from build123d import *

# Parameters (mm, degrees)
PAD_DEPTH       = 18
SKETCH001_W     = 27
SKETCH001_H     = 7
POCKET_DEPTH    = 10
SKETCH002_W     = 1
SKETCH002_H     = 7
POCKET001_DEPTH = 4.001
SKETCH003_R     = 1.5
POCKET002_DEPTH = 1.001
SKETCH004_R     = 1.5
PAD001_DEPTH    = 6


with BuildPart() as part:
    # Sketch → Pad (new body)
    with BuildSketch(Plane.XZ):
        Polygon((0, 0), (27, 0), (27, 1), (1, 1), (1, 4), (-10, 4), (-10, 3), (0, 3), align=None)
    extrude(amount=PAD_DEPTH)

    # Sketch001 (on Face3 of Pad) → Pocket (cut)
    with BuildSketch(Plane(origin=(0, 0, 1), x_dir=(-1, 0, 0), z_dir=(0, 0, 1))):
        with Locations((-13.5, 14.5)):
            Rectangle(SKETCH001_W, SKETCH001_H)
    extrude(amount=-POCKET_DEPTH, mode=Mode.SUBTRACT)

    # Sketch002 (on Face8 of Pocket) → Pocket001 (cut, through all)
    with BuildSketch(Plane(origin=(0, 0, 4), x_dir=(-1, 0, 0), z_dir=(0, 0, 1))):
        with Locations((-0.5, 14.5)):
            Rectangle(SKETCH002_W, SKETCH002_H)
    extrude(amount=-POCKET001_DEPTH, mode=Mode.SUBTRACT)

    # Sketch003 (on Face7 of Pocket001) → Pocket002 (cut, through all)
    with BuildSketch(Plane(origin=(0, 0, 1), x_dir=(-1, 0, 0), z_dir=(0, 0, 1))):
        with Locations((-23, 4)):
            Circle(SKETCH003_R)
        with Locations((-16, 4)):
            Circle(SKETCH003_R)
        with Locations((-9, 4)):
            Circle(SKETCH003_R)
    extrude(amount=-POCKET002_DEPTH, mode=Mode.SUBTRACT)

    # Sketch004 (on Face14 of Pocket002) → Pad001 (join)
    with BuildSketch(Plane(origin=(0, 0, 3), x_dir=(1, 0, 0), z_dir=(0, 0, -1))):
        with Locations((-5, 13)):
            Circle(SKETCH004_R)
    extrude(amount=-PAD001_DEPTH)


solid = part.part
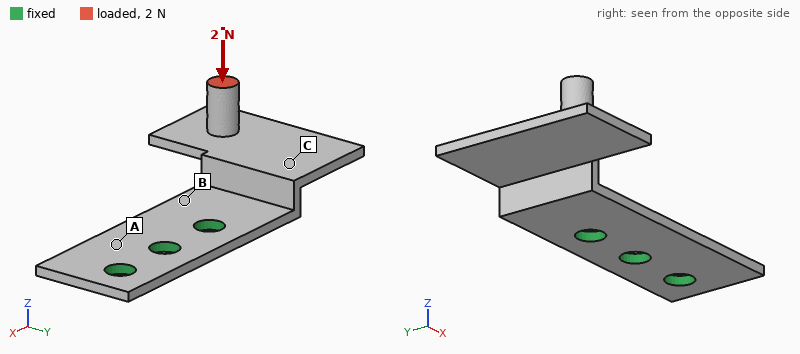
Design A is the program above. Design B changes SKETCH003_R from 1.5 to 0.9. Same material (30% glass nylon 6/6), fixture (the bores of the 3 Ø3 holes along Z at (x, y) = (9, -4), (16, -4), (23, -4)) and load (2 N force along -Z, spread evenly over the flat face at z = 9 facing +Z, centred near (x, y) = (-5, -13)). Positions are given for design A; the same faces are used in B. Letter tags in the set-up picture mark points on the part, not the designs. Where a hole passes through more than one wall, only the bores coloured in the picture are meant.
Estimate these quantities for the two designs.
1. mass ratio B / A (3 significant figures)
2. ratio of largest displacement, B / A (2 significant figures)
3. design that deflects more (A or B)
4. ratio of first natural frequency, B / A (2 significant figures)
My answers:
1.03
1.1
B
0.93
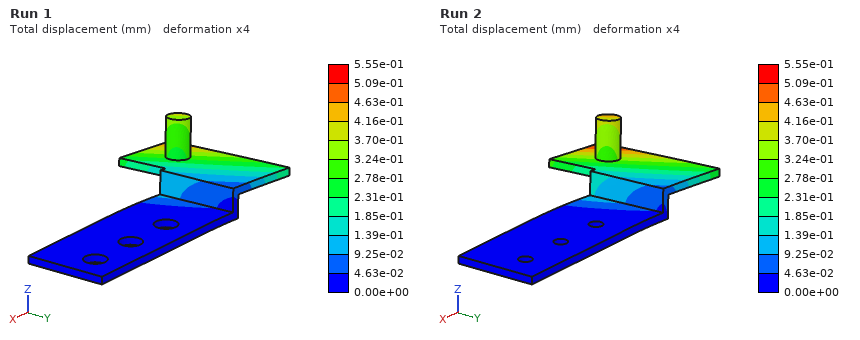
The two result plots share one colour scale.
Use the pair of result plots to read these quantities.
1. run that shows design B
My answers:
Run 2
